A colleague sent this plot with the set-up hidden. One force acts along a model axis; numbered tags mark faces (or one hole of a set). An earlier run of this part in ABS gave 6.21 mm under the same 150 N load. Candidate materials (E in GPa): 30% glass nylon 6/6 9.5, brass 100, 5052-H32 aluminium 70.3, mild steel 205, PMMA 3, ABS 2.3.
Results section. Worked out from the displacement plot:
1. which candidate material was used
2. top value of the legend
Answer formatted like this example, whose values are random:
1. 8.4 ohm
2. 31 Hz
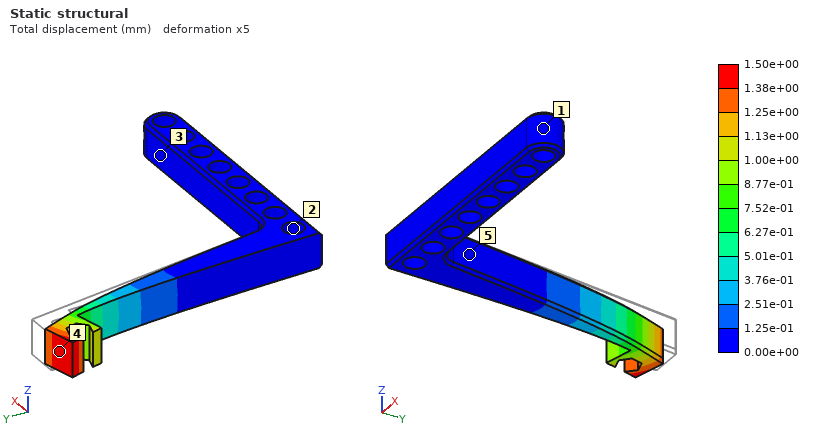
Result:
1. 30% glass nylon 6/6
2. 1.50e+00 mm
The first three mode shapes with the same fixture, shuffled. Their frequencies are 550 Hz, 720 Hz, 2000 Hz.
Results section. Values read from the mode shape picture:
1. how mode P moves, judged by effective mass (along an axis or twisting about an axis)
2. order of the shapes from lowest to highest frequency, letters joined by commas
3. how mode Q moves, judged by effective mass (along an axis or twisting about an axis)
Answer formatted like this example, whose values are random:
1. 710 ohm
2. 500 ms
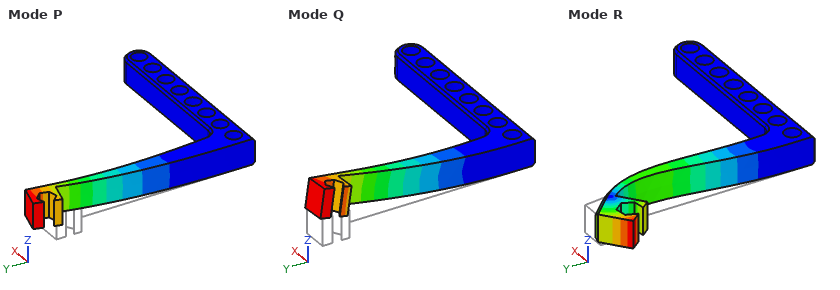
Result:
1. along X
2. P, Q, R
3. along Z
